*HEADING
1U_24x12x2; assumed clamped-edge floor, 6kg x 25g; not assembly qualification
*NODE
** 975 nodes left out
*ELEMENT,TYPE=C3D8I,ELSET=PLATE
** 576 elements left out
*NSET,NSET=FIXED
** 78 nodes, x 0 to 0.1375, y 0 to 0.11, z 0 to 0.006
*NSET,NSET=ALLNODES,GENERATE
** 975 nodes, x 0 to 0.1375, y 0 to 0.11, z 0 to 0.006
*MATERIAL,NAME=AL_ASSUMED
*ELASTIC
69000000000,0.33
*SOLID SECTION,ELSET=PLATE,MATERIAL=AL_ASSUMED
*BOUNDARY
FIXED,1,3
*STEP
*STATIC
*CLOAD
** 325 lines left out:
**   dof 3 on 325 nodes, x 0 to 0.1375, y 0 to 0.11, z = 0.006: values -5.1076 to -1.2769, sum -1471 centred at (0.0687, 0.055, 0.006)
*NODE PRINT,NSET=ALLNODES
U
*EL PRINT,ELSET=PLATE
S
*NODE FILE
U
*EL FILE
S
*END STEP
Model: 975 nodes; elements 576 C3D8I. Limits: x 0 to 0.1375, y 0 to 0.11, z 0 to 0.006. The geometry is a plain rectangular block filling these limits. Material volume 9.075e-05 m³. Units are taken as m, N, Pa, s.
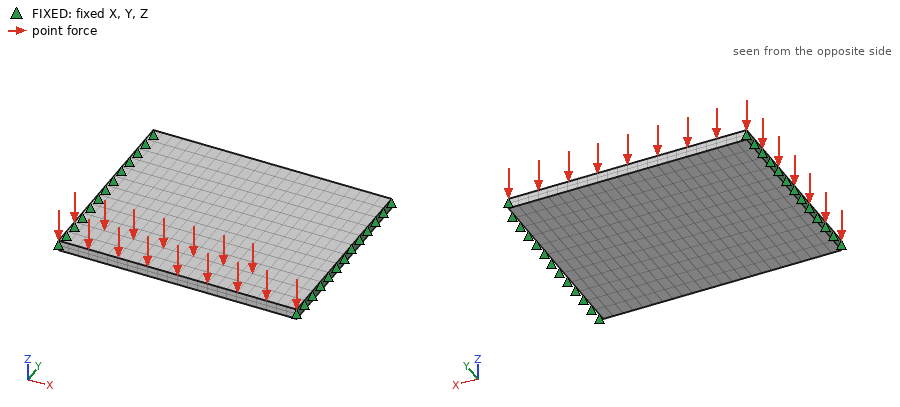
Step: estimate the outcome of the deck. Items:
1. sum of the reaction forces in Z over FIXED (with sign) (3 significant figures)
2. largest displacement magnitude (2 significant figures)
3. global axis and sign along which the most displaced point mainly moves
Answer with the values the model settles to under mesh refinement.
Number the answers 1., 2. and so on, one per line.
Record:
1. 1470 N
2. 7.5e-05 m
3. -Z
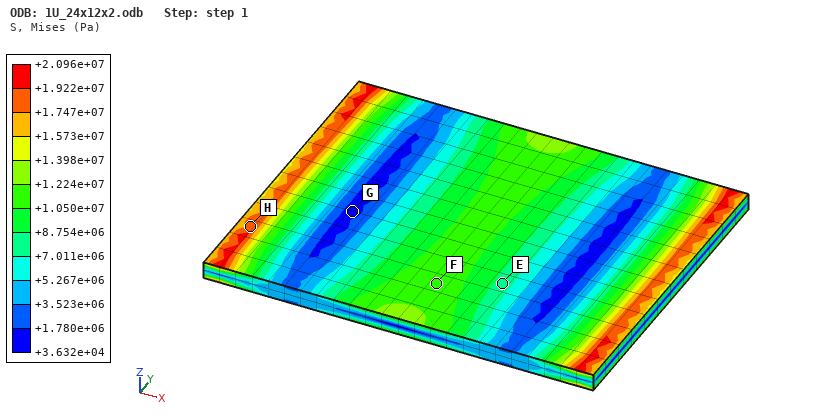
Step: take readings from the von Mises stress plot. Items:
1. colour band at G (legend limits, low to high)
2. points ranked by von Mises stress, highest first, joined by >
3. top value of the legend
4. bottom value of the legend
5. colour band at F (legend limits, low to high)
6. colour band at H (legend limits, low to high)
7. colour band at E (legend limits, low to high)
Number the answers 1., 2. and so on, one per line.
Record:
1. +3.632e+04 to +1.780e+06 Pa
2. H > F > E > G
3. +2.096e+07 Pa
4. +3.632e+04 Pa
5. +1.050e+07 to +1.224e+07 Pa
6. +1.747e+07 to +1.922e+07 Pa
7. +7.011e+06 to +8.754e+06 Pa
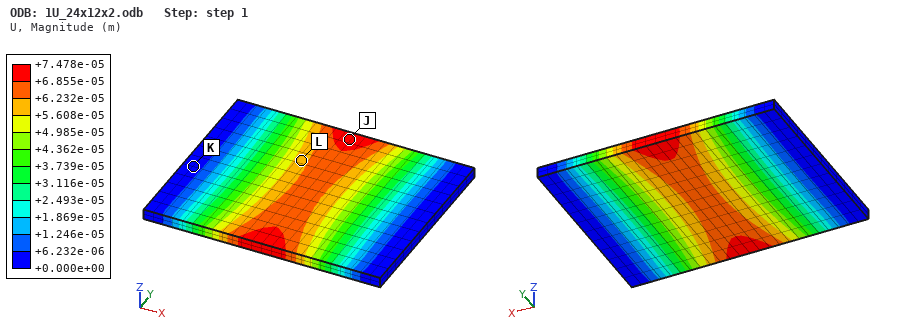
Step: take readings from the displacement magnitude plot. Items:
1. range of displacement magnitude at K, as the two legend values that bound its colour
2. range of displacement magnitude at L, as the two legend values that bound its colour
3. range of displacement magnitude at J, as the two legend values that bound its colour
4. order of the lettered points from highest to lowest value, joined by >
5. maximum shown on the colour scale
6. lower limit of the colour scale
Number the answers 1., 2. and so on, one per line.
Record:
1. +0.000e+00 to +6.232e-06 m
2. +5.608e-05 to +6.232e-05 m
3. +6.855e-05 to +7.478e-05 m
4. J > L > K
5. +7.478e-05 m
6. +0.000e+00 m
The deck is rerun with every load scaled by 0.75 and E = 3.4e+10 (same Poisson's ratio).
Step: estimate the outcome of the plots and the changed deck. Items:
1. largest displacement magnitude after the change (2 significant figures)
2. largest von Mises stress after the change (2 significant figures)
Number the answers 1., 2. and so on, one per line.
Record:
1. 1.1e-04 m
2. 1.6e+07 Pa
